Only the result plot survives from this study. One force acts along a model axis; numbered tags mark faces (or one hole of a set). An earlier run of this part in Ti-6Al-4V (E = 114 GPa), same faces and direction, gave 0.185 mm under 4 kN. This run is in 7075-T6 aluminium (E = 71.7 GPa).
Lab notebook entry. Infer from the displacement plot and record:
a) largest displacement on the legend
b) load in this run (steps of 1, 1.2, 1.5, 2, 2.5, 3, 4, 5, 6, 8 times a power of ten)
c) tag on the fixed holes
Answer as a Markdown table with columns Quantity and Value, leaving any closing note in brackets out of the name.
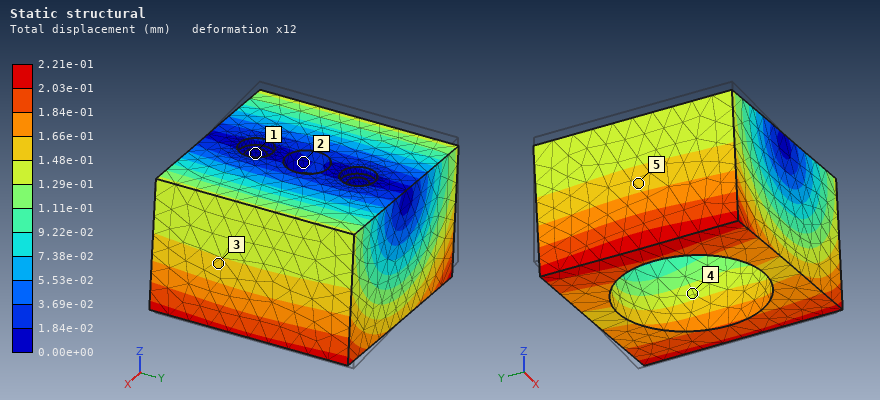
| Quantity | Value |
|---|---|
| largest displacement on the legend | 2.21e-01 mm |
| load in this run | 3 kN |
| tag on the fixed holes | 1 |
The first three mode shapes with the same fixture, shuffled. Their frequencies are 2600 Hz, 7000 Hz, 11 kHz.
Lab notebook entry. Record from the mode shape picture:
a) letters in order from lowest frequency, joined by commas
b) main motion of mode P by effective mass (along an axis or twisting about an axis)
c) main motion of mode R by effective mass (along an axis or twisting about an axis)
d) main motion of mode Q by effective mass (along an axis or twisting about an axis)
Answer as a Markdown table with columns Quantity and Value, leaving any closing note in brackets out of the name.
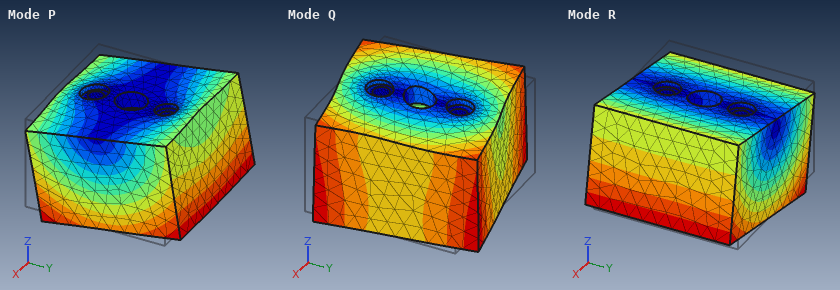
| Quantity | Value |
|---|---|
| letters in order from lowest frequency, joined by commas | R, P, Q |
| main motion of mode P by effective mass | along Y |
| main motion of mode R by effective mass | along X |
| main motion of mode Q by effective mass | twisting about Z |
